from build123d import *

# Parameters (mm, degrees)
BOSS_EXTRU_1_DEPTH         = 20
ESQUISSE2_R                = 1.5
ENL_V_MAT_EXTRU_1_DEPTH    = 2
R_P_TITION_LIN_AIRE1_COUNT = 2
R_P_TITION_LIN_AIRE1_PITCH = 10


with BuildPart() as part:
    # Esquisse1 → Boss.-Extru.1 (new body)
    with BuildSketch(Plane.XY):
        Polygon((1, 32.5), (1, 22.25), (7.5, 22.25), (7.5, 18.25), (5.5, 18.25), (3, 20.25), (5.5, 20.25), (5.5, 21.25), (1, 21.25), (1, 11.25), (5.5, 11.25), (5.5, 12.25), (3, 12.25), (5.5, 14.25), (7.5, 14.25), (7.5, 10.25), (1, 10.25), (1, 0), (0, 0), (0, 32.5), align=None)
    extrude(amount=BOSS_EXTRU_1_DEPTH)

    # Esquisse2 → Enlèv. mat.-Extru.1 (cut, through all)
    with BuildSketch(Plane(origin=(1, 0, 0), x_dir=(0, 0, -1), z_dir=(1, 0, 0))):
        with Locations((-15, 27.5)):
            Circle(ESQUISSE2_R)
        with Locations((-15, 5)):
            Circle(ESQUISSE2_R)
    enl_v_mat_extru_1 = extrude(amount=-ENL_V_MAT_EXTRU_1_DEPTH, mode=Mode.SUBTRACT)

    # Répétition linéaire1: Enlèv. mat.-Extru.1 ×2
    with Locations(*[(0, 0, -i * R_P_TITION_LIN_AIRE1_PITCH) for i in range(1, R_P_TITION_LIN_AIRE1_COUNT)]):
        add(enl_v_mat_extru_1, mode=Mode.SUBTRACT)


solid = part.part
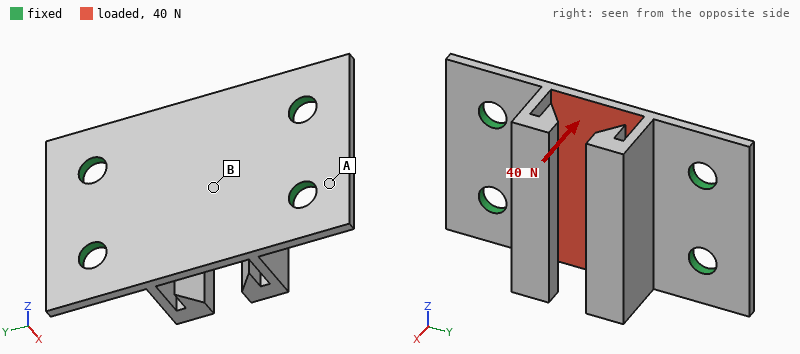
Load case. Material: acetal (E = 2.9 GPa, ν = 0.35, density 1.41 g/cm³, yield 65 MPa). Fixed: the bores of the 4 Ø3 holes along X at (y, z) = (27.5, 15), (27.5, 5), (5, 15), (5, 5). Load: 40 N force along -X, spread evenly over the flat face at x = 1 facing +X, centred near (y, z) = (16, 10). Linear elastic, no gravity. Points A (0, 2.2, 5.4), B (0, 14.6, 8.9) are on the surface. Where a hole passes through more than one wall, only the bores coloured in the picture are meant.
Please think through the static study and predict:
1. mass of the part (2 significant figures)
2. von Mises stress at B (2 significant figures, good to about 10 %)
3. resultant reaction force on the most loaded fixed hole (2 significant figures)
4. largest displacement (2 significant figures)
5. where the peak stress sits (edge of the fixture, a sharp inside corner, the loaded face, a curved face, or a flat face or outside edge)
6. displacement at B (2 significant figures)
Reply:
1.7 g
15 MPa
10 N
0.44 mm
a flat face or outside edge
0.29 mm
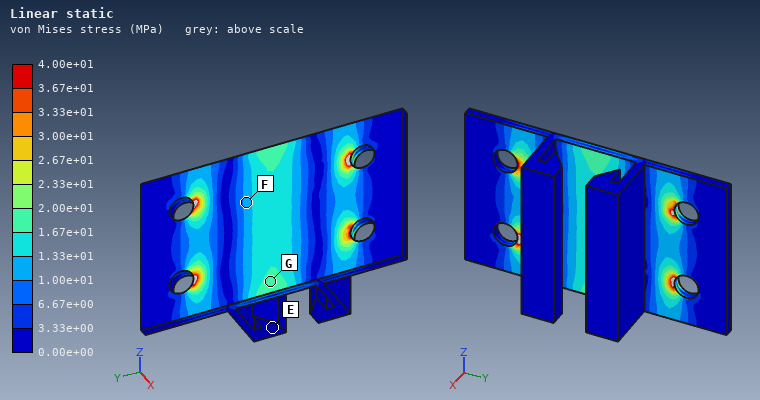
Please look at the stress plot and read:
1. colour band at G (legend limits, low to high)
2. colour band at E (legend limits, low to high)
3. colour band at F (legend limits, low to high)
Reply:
1.67e+01 to 2.00e+01 MPa
0.00e+00 to 3.33e+00 MPa
1.00e+01 to 1.33e+01 MPa
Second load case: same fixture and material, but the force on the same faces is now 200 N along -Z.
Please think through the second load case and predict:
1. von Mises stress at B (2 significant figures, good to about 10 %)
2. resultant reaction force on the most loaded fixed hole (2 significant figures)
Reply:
3.2 MPa
57 N
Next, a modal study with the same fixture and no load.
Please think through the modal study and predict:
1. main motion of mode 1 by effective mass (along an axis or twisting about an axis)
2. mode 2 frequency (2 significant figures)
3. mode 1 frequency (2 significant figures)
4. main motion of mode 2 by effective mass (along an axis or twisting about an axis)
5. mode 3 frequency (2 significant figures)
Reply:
along X
2000 Hz
1400 Hz
along Y
2400 Hz
